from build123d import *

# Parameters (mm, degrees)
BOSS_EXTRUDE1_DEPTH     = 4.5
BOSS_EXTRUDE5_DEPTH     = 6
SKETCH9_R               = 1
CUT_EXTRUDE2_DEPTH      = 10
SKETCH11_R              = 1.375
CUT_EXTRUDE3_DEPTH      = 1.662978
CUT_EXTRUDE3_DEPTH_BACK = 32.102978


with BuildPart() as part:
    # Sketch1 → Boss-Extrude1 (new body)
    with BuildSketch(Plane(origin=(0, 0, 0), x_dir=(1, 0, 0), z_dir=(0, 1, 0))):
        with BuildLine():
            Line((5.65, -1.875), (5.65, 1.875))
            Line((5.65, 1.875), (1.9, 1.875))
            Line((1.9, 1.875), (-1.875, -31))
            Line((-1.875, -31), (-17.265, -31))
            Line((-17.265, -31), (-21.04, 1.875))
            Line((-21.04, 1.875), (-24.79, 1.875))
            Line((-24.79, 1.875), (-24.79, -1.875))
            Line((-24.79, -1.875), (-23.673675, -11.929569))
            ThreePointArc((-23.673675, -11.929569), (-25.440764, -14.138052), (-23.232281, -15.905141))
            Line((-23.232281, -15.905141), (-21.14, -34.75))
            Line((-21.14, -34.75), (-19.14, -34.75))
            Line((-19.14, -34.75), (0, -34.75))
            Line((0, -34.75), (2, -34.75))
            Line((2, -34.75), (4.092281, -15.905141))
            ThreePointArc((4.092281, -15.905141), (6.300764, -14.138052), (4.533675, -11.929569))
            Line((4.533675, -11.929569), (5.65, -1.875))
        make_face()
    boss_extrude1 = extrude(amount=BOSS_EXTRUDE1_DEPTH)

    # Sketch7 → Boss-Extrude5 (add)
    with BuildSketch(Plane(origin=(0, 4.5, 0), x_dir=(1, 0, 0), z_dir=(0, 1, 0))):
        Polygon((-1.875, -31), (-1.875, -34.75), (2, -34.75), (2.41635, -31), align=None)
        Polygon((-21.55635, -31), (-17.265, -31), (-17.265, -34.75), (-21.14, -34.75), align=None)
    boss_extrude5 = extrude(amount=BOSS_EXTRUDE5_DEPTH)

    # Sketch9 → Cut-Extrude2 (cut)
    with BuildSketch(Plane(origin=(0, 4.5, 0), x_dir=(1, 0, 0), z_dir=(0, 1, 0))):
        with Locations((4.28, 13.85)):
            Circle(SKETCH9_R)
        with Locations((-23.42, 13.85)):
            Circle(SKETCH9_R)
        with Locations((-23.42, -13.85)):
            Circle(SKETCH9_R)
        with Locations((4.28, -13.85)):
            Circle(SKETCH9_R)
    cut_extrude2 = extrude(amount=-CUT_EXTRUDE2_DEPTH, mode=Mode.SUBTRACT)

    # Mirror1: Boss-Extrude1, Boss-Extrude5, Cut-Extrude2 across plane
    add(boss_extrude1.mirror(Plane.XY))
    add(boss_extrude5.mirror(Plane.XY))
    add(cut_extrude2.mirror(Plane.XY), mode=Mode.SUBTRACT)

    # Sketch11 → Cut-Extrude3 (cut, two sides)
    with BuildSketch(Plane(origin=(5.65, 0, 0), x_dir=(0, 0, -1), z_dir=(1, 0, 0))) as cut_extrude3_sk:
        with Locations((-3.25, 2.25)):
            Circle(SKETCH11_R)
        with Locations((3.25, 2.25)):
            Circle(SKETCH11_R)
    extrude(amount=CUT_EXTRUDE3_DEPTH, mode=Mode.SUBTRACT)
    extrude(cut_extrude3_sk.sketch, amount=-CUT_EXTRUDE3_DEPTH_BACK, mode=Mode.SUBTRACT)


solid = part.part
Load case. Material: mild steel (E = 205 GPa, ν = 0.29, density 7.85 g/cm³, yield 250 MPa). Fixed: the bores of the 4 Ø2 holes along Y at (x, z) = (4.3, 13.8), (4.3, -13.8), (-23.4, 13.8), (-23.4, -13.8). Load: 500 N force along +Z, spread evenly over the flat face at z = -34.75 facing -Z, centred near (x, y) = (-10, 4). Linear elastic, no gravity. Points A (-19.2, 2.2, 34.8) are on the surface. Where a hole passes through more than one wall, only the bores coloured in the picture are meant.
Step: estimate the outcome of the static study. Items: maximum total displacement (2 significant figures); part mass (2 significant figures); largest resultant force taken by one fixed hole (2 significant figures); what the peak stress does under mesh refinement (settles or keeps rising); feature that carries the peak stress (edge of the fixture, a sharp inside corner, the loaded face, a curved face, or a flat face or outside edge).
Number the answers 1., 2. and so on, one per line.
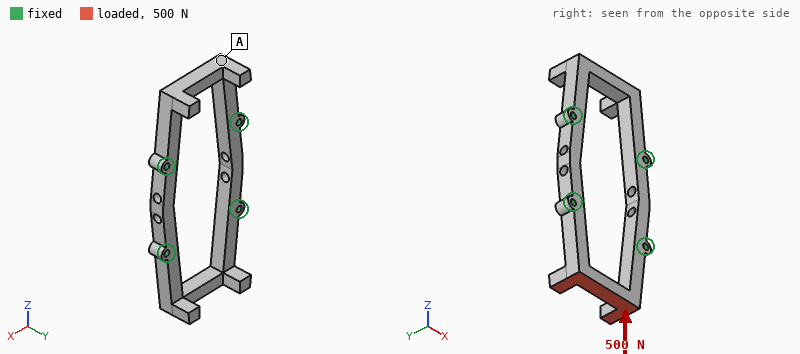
1. 19 µm
2. 27 g
3. 250 N
4. keeps rising
5. edge of the fixture
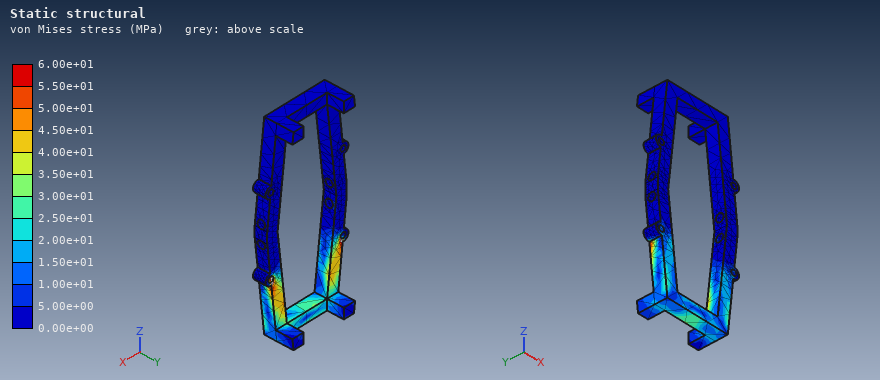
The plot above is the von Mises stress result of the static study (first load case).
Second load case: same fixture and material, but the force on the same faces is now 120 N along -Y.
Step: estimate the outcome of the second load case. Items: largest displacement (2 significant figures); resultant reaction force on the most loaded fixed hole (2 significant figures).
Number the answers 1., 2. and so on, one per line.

1. 35 µm
2. 65 N
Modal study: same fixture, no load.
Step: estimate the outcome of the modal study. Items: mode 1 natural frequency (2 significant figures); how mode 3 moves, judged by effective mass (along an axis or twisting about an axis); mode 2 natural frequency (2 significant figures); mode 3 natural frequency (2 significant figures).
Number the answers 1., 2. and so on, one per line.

1. 4700 Hz
2. along X
3. 4700 Hz
4. 7600 Hz
